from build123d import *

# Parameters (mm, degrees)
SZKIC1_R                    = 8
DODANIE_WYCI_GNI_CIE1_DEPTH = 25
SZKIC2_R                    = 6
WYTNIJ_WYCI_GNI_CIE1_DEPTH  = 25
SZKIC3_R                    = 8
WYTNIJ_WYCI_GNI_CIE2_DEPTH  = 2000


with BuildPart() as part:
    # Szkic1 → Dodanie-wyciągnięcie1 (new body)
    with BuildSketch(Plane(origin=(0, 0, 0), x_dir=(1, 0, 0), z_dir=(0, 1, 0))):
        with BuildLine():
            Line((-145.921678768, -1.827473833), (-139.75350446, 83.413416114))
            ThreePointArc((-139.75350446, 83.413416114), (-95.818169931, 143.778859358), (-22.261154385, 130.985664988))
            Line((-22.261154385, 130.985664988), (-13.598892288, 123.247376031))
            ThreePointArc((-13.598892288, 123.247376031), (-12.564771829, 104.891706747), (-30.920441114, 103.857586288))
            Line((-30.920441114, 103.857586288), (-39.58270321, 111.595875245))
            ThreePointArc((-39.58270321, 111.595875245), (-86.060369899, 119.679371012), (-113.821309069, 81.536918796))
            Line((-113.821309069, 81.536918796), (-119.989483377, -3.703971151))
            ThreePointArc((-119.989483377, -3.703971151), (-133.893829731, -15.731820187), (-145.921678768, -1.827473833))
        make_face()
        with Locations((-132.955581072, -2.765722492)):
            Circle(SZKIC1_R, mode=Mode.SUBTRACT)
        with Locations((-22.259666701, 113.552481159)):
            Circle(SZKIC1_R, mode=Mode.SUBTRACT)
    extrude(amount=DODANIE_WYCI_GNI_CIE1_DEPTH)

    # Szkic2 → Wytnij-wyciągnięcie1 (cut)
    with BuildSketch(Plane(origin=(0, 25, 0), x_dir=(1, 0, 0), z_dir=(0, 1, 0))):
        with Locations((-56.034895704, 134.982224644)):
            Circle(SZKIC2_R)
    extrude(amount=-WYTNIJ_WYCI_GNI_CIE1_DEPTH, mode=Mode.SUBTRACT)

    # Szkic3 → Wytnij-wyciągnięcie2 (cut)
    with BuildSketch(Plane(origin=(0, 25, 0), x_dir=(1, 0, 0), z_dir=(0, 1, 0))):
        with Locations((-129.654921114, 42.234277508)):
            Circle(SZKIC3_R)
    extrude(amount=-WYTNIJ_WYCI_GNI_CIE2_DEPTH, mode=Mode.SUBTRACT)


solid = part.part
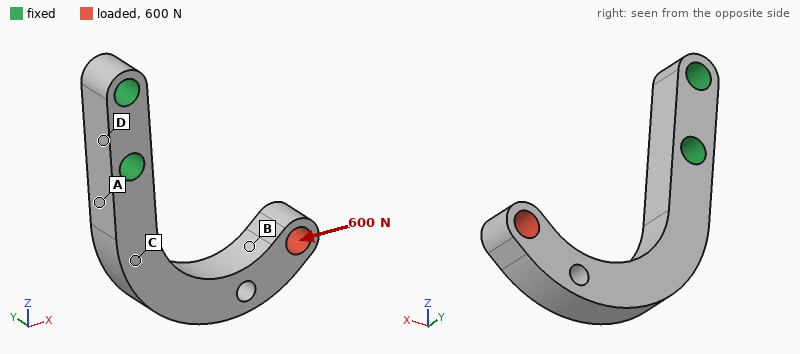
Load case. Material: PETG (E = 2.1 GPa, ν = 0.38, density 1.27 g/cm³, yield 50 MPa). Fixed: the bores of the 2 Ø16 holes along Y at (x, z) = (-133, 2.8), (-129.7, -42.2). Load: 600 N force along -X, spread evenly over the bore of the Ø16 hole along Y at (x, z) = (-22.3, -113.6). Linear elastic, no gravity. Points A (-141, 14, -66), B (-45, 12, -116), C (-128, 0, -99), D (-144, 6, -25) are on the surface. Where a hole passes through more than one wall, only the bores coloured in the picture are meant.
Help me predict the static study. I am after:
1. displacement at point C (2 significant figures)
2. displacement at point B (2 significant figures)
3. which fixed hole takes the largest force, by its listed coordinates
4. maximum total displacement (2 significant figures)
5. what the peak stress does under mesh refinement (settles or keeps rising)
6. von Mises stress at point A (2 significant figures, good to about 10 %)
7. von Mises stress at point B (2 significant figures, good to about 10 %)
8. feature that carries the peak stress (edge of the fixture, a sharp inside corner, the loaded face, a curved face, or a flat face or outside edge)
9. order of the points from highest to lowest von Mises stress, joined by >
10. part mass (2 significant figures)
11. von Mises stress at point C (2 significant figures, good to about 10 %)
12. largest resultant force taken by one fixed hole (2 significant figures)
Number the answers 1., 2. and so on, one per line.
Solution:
1. 0.67 mm
2. 1.8 mm
3. (-129.7, -42.2)
4. 2.0 mm
5. keeps rising
6. 10 MPa
7. 4.6 MPa
8. edge of the fixture
9. A > B > C > D
10. 180 g
11. 2.8 MPa
12. 670 N
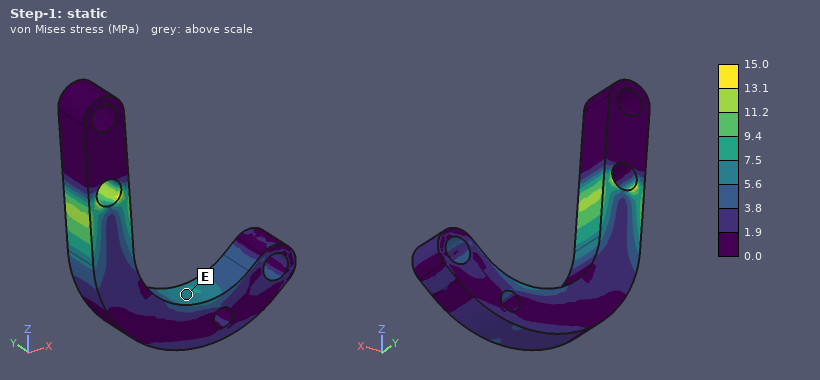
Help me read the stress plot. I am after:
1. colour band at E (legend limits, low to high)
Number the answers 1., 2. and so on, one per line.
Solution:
1. 5.6 to 7.5 MPa
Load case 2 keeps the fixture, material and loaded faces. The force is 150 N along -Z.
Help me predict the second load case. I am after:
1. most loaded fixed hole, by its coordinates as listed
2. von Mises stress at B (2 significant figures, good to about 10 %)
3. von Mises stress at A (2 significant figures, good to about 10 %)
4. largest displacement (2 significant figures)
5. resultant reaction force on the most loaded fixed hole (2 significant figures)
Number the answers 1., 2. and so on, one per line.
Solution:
1. (-129.7, -42.2)
2. 0.67 MPa
3. 5.4 MPa
4. 2.5 mm
5. 150 N
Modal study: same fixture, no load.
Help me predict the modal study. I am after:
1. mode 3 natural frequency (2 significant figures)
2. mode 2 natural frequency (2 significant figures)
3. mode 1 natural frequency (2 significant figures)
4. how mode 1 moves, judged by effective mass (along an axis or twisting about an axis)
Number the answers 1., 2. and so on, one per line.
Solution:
1. 520 Hz
2. 190 Hz
3. 180 Hz
4. along Y
